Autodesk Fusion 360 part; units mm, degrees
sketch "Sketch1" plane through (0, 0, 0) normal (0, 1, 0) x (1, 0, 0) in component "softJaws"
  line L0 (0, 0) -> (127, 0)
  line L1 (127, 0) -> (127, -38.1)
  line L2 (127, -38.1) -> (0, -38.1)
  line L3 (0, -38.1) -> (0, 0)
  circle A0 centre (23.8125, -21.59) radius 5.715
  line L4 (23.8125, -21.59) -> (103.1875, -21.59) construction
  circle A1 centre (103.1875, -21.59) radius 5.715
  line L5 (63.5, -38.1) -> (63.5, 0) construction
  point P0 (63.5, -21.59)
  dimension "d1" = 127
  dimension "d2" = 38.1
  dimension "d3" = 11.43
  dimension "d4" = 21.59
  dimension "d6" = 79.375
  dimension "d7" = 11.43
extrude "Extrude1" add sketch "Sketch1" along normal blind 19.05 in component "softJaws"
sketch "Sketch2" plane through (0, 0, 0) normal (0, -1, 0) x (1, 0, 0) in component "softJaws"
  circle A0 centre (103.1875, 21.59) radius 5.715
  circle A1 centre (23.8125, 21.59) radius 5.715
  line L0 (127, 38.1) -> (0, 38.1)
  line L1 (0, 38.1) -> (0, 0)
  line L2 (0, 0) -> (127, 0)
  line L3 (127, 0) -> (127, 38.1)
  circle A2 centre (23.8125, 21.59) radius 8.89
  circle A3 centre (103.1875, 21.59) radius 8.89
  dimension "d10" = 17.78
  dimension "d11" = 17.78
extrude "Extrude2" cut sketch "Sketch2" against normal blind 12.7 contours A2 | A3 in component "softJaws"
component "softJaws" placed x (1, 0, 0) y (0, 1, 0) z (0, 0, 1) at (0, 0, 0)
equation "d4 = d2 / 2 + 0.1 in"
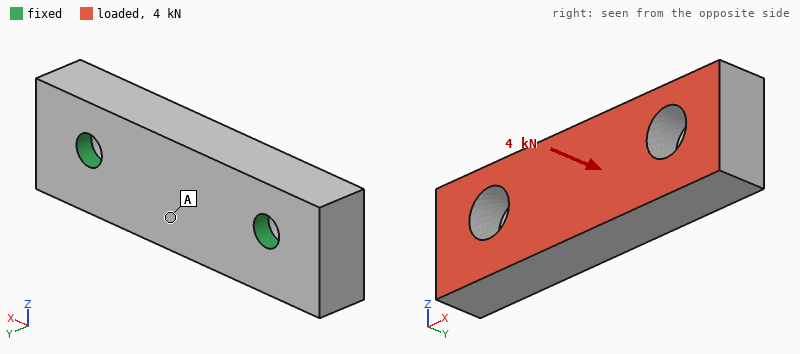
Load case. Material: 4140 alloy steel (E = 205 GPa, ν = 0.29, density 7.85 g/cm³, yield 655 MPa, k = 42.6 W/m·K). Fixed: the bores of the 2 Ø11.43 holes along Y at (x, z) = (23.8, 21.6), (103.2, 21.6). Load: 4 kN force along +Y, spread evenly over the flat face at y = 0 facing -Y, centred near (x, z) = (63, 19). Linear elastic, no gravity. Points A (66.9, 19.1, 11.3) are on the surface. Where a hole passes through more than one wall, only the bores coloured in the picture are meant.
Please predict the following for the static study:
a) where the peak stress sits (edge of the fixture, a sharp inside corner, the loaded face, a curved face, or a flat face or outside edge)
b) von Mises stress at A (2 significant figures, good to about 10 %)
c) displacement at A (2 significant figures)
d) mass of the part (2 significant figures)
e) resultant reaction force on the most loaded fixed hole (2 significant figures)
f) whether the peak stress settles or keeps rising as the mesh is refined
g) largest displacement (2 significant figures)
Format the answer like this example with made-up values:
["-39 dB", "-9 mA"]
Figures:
["edge of the fixture", "4.1 MPa", "2.6 µm", "660 g", "2.1 kN", "keeps rising", "3.5 µm"]
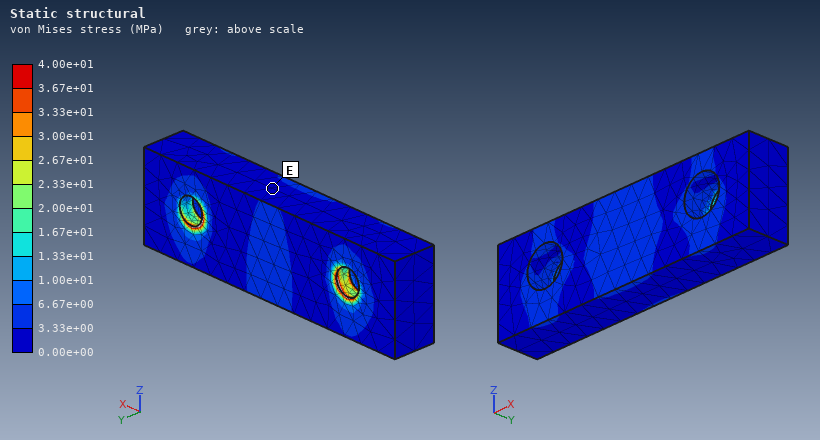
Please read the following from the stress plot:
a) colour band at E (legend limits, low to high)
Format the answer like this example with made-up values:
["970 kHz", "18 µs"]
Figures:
["0.00e+00 to 3.33e+00 MPa"]
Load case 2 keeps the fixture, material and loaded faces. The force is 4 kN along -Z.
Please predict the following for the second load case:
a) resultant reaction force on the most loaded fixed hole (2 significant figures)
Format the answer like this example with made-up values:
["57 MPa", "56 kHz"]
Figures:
["2.0 kN"]
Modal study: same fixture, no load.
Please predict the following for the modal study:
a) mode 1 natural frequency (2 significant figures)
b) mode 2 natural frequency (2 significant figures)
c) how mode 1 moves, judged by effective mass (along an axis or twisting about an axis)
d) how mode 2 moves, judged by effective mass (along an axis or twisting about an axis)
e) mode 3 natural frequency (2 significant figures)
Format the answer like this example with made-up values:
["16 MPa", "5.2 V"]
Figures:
["6100 Hz", "8600 Hz", "along Z", "along Y", "10 kHz"]
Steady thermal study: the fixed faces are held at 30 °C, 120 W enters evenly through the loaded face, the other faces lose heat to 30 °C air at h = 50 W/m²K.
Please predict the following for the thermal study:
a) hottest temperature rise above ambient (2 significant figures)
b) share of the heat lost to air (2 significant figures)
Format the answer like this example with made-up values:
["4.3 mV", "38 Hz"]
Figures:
["48 K", "15 %"]
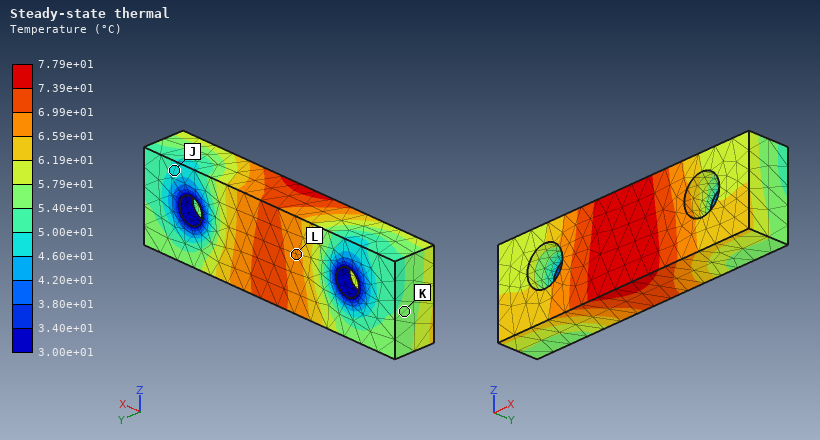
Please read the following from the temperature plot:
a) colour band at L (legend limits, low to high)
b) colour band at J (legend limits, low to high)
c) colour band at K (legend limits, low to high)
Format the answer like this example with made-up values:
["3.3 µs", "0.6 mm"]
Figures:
["6.59e+01 to 6.99e+01 °C", "4.60e+01 to 5.00e+01 °C", "5.40e+01 to 5.79e+01 °C"]
